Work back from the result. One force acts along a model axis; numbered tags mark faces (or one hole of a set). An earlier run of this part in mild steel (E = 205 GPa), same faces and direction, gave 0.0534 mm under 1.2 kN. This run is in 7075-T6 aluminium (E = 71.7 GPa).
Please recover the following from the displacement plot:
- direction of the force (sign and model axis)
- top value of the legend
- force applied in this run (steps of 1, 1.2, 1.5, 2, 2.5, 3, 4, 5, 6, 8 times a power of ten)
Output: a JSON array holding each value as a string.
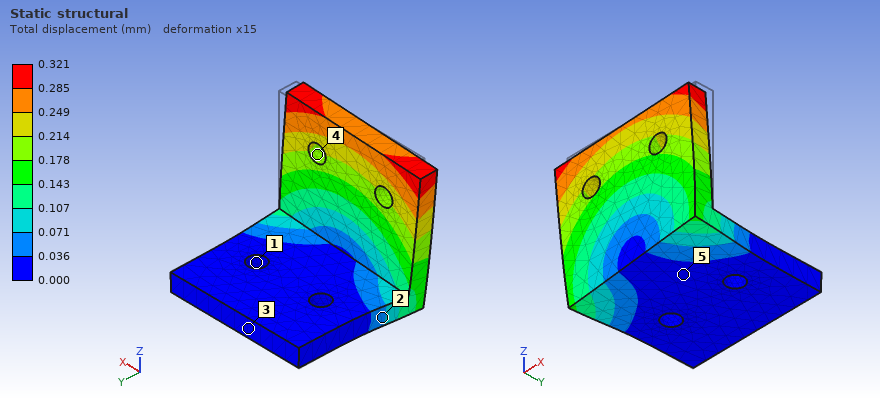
["-X", "0.321 mm", "2.5 kN"]
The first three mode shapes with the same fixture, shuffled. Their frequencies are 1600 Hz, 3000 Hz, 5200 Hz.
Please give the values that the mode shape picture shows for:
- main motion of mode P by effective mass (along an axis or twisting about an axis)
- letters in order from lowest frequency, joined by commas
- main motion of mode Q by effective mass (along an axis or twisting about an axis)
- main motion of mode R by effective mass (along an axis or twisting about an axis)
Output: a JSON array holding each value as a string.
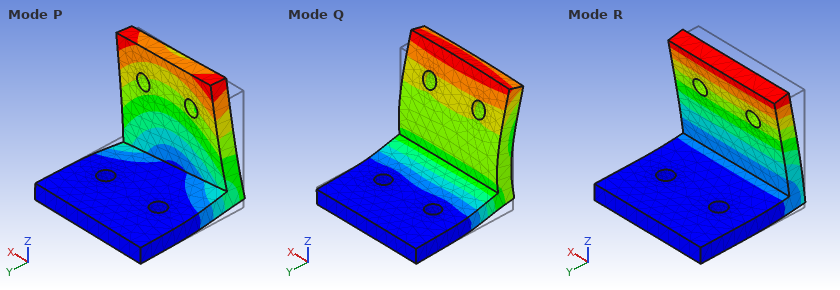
["along X", "R, P, Q", "along Z", "along Y"]
